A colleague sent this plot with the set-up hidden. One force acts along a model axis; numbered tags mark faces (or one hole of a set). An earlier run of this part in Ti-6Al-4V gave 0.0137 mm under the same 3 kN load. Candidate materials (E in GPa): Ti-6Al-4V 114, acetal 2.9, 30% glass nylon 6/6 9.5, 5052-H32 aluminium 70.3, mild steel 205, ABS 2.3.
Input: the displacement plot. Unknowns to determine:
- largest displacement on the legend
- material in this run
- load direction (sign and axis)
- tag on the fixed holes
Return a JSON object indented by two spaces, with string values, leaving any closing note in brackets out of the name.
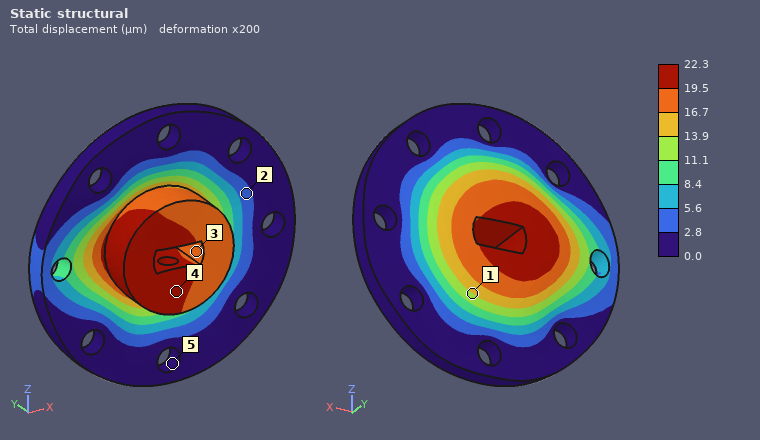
{
  "largest displacement on the legend": "22.3 µm",
  "material in this run": "5052-H32 aluminium",
  "load direction": "+Y",
  "tag on the fixed holes": "5"
}
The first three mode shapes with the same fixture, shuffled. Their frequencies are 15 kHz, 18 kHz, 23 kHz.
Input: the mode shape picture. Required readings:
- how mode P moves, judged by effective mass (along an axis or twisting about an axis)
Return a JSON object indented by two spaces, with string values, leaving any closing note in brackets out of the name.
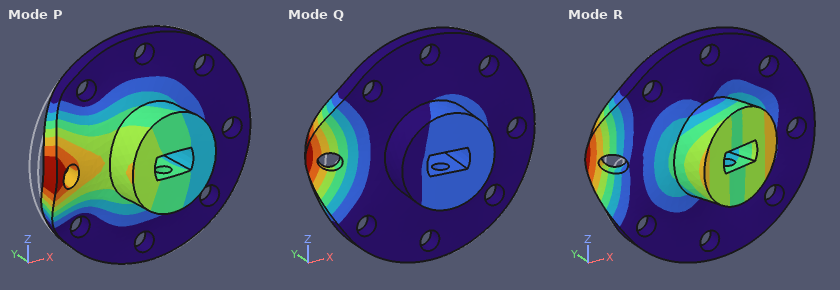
{
  "how mode P moves, judged by effective mass": "along Y"
}
